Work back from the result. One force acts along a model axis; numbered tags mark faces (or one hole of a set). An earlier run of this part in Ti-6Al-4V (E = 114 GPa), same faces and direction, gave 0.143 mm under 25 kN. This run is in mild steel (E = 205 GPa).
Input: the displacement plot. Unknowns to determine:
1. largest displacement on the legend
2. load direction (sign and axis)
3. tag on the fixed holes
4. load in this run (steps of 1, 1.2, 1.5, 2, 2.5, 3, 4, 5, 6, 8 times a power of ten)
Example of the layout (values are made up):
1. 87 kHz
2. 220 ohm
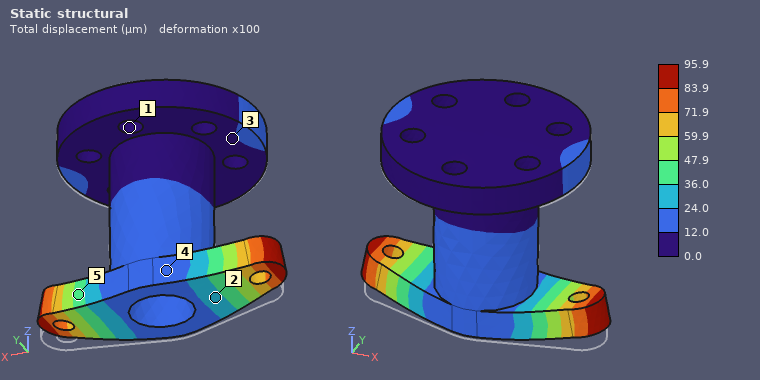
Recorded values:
1. 95.9 µm
2. +Z
3. 1
4. 30 kN
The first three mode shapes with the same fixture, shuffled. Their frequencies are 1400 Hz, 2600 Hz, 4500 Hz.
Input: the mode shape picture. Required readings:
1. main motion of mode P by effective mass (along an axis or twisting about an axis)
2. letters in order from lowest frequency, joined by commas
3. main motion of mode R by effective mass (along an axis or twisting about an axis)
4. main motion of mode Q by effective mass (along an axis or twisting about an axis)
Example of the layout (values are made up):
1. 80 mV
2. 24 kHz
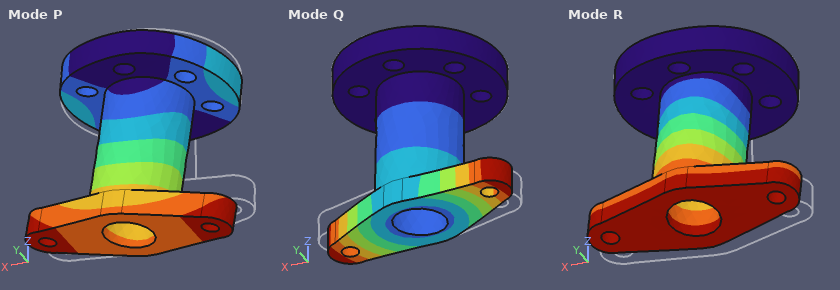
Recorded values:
1. along X
2. P, R, Q
3. along Y
4. twisting about Z
